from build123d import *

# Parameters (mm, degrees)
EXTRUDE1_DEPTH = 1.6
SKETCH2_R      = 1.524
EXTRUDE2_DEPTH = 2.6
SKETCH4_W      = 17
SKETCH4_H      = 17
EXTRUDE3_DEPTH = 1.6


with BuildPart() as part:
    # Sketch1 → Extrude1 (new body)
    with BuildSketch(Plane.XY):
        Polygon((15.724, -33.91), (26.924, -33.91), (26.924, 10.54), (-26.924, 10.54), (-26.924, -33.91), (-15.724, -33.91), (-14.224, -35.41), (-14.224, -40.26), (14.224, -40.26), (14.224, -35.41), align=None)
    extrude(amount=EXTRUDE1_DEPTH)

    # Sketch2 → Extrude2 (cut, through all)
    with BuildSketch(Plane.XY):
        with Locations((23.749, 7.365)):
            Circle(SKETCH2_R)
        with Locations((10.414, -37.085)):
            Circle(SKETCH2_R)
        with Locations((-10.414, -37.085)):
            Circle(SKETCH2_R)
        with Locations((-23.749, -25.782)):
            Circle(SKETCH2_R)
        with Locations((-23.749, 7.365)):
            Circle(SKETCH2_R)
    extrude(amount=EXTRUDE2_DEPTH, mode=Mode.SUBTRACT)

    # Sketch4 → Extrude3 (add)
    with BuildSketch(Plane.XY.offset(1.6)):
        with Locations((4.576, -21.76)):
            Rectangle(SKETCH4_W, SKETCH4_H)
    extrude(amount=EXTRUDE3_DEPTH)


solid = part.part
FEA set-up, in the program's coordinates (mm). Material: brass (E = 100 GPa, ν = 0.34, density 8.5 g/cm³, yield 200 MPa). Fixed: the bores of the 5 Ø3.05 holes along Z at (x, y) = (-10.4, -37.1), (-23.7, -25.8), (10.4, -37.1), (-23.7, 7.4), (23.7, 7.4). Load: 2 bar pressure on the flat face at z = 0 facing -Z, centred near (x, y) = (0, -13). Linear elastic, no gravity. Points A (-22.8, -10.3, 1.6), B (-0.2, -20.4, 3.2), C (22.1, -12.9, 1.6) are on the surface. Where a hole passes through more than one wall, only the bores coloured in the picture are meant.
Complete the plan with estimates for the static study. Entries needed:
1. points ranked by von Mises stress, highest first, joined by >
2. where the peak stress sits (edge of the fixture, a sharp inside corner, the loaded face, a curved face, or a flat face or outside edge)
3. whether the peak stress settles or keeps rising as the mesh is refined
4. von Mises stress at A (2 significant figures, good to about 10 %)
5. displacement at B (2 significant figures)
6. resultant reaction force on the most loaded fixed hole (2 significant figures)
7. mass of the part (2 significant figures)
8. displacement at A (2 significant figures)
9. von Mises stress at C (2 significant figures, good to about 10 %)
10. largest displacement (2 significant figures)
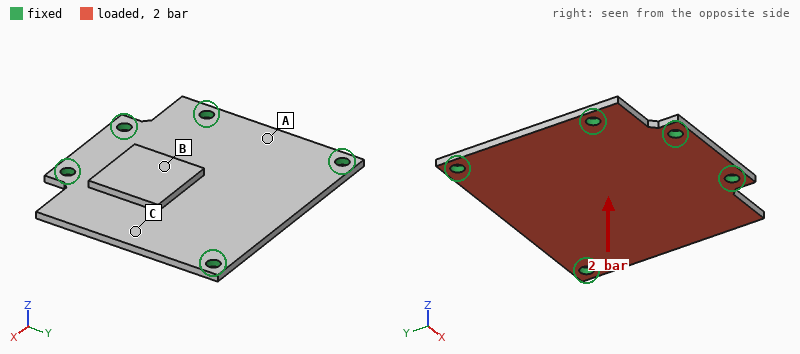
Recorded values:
C > A > B
edge of the fixture
keeps rising
28 MPa
59 µm
140 N
38 g
26 µm
51 MPa
99 µm
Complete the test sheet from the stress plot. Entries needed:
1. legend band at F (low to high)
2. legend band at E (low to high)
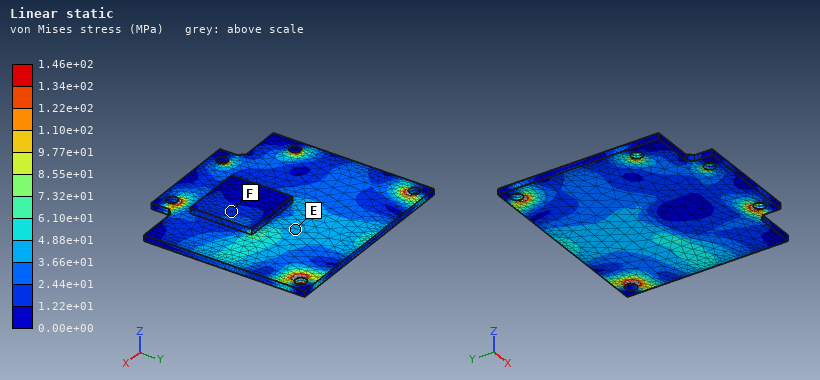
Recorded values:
1.22e+01 to 2.44e+01 MPa
3.66e+01 to 4.88e+01 MPa
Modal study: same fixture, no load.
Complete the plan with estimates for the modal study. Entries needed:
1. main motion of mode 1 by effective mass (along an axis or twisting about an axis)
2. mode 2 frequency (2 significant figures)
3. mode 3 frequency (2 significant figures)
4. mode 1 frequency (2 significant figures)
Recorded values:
along Z
3000 Hz
4300 Hz
2200 Hz
